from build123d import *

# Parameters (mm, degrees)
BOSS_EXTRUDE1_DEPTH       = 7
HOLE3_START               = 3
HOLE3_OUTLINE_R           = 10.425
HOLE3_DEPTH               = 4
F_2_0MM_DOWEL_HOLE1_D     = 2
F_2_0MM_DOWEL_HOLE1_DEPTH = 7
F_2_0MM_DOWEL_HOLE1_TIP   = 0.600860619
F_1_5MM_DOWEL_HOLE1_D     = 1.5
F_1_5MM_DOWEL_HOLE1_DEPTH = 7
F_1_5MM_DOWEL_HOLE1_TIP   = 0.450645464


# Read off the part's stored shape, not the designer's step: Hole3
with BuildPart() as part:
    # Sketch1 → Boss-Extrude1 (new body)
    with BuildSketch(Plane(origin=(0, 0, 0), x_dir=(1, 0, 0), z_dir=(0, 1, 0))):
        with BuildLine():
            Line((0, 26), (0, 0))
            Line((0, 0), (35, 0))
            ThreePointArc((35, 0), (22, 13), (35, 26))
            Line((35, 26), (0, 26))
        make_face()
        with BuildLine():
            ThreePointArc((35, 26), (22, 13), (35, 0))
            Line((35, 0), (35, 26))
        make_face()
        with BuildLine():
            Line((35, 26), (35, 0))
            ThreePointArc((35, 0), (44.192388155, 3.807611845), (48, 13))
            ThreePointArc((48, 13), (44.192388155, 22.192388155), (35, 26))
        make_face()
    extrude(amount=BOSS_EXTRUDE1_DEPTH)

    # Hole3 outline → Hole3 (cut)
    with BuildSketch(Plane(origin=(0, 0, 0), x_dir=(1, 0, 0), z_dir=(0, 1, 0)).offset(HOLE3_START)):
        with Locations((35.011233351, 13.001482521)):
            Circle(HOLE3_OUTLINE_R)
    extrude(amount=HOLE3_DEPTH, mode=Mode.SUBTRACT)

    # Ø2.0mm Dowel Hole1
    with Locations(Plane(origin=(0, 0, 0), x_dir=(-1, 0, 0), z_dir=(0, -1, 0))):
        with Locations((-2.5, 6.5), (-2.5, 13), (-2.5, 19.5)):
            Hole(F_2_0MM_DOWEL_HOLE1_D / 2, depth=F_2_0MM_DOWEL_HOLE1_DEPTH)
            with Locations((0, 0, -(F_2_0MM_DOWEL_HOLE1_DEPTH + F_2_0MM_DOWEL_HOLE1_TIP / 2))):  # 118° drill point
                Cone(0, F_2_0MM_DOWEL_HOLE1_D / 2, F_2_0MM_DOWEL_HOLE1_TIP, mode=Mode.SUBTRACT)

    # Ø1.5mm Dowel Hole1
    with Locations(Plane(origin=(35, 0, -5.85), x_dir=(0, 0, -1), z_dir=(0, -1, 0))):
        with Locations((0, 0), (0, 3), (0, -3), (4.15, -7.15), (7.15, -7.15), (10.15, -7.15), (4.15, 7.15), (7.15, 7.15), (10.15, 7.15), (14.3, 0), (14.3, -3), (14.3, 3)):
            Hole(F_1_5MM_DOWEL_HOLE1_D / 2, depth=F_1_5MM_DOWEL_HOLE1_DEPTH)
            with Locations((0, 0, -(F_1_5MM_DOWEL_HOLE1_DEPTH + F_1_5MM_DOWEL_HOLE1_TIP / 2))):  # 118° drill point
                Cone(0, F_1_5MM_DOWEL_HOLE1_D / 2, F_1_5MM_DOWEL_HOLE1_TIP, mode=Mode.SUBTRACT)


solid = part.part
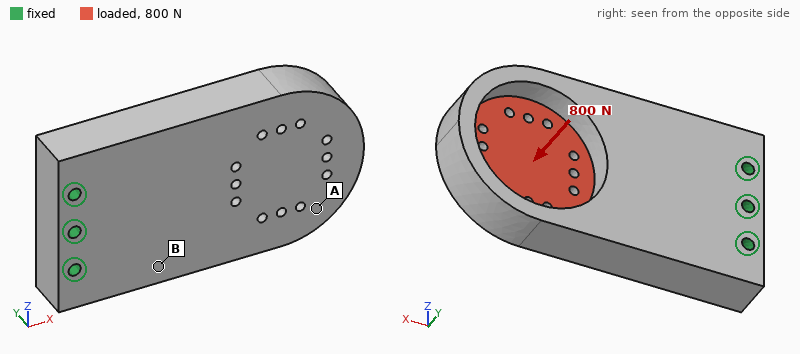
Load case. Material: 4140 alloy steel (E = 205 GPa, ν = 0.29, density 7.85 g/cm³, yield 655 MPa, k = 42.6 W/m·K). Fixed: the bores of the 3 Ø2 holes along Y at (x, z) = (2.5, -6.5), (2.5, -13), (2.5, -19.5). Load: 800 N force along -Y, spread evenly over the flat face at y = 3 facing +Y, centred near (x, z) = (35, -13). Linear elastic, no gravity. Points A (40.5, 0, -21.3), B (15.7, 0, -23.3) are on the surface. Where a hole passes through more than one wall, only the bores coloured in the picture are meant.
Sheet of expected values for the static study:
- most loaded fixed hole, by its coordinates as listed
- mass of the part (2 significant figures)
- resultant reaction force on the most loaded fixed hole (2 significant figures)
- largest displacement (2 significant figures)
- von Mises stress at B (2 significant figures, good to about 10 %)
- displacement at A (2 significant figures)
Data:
(2.5, -13)
53 g
480 N
0.12 mm
72 MPa
0.092 mm
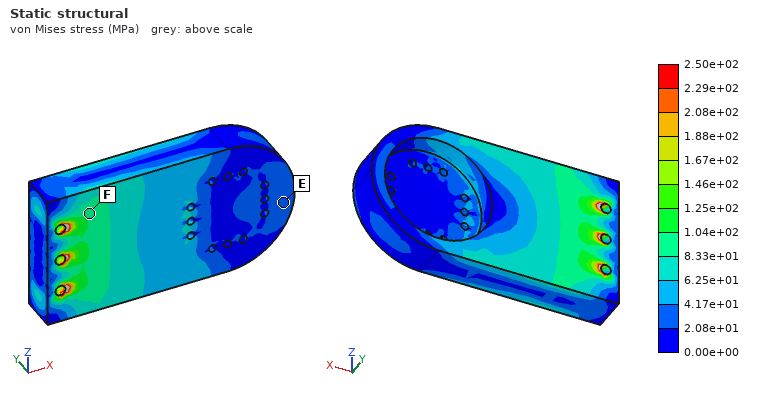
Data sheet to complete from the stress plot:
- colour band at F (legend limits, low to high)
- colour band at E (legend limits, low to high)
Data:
8.33e+01 to 1.04e+02 MPa
2.08e+01 to 4.17e+01 MPa
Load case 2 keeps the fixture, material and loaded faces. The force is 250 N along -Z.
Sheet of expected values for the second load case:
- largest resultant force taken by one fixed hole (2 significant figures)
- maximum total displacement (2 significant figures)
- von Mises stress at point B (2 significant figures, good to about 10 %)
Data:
560 N
5.5 µm
6.1 MPa
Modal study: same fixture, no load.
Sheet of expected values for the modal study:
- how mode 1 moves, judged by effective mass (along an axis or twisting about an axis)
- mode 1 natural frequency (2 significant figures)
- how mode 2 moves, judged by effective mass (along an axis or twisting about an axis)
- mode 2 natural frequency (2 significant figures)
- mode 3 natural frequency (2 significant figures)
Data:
along Y
3500 Hz
along Z
8500 Hz
9700 Hz
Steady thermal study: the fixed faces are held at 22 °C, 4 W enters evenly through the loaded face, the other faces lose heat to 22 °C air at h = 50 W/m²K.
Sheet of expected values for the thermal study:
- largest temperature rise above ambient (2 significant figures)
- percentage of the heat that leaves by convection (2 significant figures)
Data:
17 K
33 %
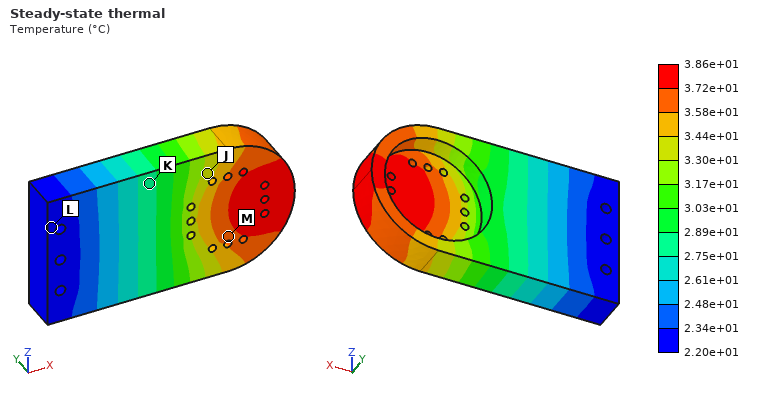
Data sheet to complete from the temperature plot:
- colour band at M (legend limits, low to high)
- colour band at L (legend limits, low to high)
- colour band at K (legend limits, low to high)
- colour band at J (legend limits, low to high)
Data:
3.58e+01 to 3.72e+01 °C
2.20e+01 to 2.34e+01 °C
2.75e+01 to 2.89e+01 °C
3.30e+01 to 3.44e+01 °C
